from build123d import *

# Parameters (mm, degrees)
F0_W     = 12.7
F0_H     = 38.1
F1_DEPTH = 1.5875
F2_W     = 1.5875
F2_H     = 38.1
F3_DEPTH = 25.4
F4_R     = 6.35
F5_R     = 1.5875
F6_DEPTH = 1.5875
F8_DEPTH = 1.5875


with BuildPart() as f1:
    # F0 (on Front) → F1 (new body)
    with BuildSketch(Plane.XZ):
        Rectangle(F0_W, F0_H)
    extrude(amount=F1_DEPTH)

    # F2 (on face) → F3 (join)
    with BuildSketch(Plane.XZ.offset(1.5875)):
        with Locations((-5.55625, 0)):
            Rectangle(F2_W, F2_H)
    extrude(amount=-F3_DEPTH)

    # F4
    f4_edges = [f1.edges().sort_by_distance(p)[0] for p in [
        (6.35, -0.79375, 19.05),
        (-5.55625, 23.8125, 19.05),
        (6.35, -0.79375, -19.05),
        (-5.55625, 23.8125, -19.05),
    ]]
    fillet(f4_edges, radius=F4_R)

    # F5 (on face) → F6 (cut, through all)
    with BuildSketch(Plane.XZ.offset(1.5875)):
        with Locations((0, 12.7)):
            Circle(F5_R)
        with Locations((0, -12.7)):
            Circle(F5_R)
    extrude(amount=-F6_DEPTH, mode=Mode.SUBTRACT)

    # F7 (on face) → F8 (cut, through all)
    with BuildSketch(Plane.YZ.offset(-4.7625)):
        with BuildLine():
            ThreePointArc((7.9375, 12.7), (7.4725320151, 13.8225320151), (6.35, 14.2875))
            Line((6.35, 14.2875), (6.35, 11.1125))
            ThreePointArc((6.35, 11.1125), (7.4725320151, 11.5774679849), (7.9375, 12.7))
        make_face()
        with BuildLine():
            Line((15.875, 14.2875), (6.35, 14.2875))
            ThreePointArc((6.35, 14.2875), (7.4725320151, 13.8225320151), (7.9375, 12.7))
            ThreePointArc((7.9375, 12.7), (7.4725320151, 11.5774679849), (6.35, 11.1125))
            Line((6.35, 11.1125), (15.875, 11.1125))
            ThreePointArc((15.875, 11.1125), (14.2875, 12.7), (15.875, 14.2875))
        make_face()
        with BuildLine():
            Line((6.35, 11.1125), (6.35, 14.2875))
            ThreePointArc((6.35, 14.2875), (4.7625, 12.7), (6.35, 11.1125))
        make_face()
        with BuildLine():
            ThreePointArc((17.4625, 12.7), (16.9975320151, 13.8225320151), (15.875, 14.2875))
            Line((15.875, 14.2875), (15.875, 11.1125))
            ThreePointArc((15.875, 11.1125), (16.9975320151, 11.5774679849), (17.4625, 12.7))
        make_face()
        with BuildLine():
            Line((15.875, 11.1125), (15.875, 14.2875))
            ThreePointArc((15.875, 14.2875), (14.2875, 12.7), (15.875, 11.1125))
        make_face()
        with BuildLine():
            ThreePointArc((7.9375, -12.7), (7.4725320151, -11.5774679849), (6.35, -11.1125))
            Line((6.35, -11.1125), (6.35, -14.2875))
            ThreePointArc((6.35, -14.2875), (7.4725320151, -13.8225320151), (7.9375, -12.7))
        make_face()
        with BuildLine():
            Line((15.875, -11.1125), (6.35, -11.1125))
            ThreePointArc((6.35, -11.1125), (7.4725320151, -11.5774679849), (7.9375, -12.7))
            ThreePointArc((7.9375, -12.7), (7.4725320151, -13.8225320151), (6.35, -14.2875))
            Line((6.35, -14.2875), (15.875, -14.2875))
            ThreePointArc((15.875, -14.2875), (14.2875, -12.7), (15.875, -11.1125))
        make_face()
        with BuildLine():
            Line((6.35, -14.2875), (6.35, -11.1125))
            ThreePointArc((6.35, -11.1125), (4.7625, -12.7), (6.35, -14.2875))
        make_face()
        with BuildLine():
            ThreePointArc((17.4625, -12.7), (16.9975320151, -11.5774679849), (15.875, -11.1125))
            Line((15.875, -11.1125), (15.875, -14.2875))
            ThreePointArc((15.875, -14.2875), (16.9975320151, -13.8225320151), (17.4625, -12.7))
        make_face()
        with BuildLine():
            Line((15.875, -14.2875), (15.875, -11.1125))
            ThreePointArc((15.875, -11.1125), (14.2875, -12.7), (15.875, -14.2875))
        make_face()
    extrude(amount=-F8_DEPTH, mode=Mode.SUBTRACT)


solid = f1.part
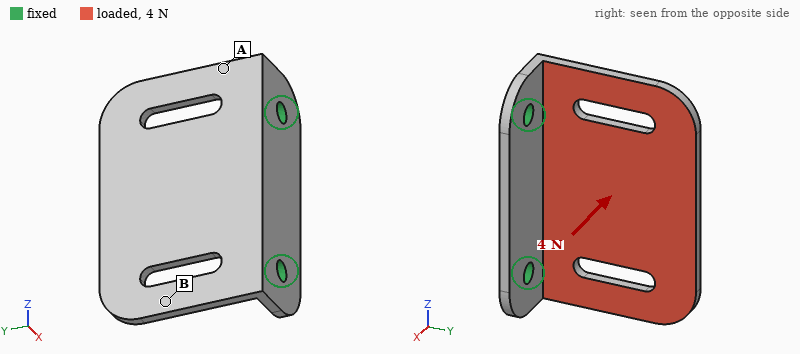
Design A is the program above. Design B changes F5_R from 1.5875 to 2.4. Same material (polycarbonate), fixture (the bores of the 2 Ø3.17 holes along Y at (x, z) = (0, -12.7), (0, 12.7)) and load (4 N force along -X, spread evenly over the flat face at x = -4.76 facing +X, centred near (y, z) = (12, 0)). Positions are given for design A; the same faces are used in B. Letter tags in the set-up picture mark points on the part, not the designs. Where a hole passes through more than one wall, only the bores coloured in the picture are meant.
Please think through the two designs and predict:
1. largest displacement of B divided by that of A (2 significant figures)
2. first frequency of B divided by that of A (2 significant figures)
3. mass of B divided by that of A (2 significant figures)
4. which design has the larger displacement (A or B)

0.89
1.1
0.98
A
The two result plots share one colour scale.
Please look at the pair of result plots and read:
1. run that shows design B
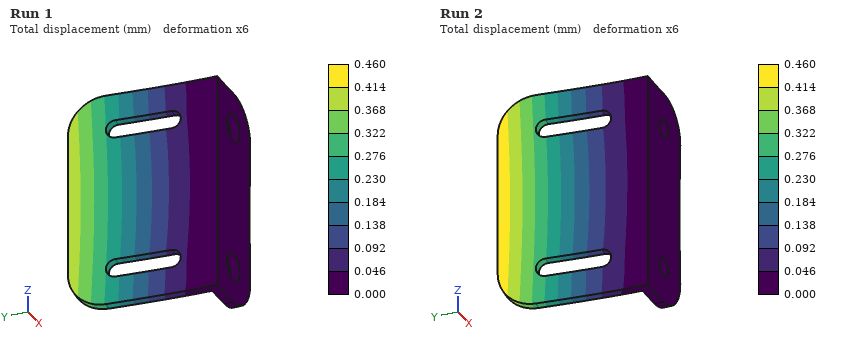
Run 1
